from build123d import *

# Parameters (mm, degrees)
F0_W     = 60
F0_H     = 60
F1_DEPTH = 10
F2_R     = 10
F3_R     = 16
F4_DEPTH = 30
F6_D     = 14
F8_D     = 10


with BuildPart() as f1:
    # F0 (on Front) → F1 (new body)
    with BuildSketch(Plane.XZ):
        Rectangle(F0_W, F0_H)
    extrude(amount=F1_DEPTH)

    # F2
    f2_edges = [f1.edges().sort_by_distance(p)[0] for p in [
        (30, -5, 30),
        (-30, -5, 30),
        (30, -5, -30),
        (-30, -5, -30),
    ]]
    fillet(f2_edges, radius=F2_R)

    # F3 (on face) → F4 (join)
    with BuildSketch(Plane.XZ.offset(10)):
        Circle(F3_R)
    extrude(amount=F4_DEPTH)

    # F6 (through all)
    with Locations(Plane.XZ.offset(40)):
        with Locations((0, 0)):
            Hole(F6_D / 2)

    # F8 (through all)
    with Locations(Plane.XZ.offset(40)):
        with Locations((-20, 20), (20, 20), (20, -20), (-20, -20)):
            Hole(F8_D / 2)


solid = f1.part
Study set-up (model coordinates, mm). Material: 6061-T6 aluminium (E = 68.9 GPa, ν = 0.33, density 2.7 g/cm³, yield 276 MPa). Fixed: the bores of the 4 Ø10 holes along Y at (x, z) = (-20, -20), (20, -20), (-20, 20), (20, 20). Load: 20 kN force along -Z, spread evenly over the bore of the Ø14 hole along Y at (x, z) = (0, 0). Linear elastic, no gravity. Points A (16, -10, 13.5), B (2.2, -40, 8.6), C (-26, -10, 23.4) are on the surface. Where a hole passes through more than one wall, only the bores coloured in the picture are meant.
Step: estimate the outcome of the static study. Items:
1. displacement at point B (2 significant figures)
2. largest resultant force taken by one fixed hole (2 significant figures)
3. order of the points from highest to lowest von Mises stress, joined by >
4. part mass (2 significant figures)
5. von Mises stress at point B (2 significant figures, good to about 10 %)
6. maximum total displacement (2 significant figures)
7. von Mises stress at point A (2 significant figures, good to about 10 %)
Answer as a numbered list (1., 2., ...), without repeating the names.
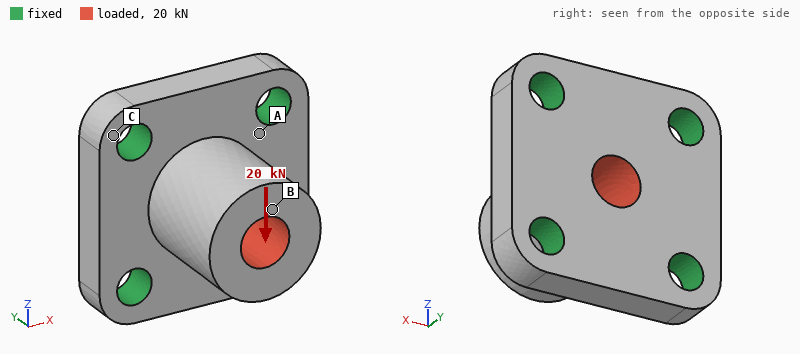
1. 82 µm
2. 7.0 kN
3. A > B > C
4. 130 g
5. 23 MPa
6. 85 µm
7. 45 MPa
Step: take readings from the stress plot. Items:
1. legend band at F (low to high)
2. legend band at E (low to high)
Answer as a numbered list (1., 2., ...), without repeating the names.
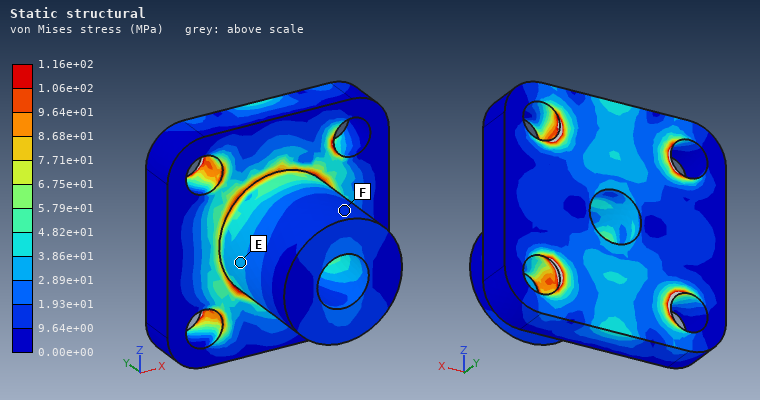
1. 9.64e+00 to 1.93e+01 MPa
2. 2.89e+01 to 3.86e+01 MPa
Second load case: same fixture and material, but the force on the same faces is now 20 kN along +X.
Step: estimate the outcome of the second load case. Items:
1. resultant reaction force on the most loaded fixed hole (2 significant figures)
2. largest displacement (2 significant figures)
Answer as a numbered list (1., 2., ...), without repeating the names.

1. 7.0 kN
2. 85 µm
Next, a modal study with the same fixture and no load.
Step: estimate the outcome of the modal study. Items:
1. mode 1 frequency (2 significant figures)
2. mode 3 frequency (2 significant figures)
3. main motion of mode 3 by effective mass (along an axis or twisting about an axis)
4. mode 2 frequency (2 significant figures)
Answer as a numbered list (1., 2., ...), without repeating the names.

1. 11 kHz
2. 17 kHz
3. along Y
4. 11 kHz
